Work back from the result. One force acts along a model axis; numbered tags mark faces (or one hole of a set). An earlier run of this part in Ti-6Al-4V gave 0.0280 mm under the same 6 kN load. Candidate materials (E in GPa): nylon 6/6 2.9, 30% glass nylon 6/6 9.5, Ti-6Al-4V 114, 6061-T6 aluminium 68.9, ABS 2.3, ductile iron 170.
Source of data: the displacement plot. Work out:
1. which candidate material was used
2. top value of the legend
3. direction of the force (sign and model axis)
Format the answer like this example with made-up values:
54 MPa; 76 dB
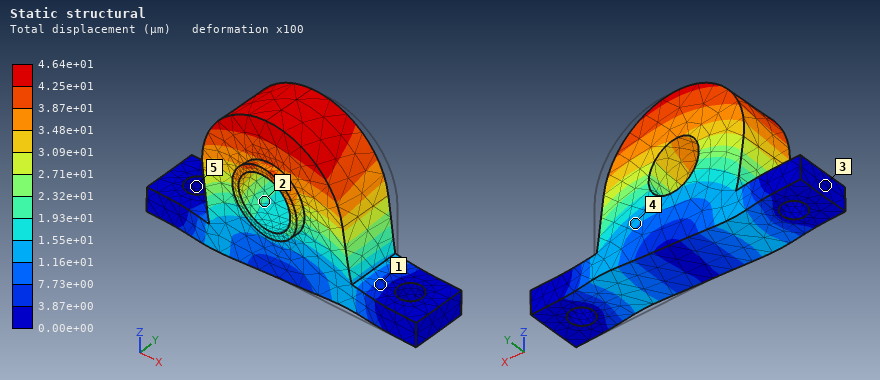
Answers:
6061-T6 aluminium; 4.64e+01 µm; -X
